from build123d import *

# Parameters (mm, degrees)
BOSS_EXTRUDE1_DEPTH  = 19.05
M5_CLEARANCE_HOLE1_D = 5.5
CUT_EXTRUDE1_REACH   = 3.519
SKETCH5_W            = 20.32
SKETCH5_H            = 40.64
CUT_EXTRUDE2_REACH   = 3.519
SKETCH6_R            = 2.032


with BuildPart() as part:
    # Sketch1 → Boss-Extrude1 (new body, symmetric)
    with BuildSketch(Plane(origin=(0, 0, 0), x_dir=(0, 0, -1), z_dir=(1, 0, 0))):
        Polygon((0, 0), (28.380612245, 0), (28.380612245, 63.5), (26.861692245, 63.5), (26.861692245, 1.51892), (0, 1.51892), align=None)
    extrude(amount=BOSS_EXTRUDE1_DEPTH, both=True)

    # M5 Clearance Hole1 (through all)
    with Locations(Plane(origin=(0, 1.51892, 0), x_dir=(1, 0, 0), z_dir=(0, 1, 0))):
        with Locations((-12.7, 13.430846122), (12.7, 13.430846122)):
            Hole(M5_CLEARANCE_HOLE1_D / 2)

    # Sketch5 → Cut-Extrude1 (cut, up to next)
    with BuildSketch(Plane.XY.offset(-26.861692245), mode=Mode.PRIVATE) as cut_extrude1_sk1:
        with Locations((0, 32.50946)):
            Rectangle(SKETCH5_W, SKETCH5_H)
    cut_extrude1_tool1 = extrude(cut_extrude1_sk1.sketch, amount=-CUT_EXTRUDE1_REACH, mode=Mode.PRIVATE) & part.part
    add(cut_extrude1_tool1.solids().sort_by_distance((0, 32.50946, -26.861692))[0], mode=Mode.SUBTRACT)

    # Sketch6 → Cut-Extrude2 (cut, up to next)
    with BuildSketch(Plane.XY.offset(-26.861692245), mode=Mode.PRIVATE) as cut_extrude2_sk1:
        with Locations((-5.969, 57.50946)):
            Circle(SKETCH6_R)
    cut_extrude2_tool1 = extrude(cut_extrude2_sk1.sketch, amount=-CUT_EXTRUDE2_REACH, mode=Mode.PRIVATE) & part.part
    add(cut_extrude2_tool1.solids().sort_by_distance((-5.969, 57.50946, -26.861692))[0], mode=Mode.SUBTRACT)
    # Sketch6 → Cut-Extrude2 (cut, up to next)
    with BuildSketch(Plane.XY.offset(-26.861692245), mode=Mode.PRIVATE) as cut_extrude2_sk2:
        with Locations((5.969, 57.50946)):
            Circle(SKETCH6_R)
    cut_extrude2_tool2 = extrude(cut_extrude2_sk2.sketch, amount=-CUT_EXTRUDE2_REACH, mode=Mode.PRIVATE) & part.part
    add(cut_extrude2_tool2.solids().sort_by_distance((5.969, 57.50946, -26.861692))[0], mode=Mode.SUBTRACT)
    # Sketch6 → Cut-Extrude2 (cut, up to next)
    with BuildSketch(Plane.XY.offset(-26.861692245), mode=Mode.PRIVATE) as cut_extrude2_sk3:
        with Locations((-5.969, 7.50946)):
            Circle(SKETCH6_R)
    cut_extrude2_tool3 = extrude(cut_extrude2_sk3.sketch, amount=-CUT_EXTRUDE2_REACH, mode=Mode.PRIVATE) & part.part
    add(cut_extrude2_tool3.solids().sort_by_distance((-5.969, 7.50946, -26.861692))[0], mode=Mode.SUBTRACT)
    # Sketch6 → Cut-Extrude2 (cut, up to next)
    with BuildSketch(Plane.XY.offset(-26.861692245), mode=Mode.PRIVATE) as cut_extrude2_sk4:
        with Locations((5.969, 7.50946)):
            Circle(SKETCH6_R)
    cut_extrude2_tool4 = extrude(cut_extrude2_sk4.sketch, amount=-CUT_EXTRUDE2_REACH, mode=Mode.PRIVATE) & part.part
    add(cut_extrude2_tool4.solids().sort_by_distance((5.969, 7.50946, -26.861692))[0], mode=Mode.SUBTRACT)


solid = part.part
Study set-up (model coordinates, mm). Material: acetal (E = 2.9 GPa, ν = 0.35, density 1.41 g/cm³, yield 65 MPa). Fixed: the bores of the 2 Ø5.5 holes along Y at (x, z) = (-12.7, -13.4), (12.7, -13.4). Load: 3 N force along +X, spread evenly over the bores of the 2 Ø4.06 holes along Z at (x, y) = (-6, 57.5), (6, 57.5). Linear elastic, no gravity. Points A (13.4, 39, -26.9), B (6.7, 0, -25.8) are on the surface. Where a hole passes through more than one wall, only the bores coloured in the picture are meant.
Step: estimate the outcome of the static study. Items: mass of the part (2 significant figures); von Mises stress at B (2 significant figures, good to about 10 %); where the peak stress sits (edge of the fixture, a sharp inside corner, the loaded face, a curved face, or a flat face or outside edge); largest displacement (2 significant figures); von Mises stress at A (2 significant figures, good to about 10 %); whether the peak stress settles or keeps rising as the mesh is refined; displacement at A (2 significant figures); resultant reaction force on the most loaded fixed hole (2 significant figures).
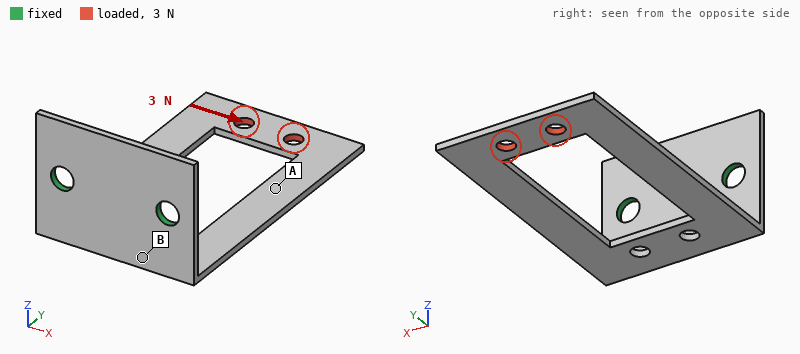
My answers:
5.4 g
3.2 MPa
edge of the fixture
0.85 mm
0.81 MPa
keeps rising
0.54 mm
6.5 N
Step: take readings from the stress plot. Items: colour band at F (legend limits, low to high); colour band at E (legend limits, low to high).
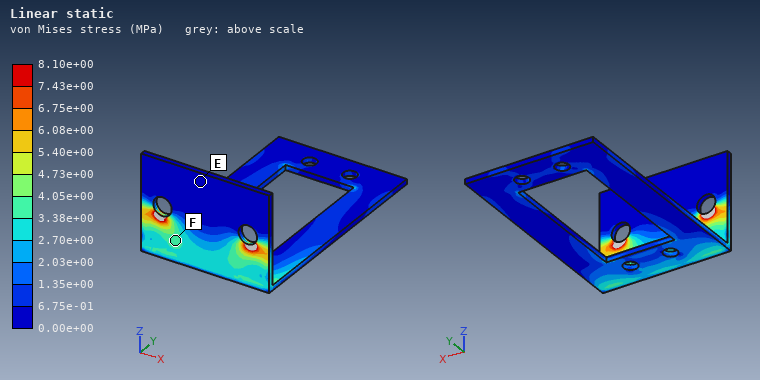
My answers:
3.38e+00 to 4.05e+00 MPa
0.00e+00 to 6.75e-01 MPa
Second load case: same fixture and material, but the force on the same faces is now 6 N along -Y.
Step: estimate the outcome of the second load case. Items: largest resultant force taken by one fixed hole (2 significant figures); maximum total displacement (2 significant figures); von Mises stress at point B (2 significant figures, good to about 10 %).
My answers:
3.0 N
0.89 mm
0.92 MPa
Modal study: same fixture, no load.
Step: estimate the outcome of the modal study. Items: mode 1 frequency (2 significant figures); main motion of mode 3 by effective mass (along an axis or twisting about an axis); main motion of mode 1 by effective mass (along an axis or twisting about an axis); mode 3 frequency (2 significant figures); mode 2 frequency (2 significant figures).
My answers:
68 Hz
along X
along Z
280 Hz
220 Hz
